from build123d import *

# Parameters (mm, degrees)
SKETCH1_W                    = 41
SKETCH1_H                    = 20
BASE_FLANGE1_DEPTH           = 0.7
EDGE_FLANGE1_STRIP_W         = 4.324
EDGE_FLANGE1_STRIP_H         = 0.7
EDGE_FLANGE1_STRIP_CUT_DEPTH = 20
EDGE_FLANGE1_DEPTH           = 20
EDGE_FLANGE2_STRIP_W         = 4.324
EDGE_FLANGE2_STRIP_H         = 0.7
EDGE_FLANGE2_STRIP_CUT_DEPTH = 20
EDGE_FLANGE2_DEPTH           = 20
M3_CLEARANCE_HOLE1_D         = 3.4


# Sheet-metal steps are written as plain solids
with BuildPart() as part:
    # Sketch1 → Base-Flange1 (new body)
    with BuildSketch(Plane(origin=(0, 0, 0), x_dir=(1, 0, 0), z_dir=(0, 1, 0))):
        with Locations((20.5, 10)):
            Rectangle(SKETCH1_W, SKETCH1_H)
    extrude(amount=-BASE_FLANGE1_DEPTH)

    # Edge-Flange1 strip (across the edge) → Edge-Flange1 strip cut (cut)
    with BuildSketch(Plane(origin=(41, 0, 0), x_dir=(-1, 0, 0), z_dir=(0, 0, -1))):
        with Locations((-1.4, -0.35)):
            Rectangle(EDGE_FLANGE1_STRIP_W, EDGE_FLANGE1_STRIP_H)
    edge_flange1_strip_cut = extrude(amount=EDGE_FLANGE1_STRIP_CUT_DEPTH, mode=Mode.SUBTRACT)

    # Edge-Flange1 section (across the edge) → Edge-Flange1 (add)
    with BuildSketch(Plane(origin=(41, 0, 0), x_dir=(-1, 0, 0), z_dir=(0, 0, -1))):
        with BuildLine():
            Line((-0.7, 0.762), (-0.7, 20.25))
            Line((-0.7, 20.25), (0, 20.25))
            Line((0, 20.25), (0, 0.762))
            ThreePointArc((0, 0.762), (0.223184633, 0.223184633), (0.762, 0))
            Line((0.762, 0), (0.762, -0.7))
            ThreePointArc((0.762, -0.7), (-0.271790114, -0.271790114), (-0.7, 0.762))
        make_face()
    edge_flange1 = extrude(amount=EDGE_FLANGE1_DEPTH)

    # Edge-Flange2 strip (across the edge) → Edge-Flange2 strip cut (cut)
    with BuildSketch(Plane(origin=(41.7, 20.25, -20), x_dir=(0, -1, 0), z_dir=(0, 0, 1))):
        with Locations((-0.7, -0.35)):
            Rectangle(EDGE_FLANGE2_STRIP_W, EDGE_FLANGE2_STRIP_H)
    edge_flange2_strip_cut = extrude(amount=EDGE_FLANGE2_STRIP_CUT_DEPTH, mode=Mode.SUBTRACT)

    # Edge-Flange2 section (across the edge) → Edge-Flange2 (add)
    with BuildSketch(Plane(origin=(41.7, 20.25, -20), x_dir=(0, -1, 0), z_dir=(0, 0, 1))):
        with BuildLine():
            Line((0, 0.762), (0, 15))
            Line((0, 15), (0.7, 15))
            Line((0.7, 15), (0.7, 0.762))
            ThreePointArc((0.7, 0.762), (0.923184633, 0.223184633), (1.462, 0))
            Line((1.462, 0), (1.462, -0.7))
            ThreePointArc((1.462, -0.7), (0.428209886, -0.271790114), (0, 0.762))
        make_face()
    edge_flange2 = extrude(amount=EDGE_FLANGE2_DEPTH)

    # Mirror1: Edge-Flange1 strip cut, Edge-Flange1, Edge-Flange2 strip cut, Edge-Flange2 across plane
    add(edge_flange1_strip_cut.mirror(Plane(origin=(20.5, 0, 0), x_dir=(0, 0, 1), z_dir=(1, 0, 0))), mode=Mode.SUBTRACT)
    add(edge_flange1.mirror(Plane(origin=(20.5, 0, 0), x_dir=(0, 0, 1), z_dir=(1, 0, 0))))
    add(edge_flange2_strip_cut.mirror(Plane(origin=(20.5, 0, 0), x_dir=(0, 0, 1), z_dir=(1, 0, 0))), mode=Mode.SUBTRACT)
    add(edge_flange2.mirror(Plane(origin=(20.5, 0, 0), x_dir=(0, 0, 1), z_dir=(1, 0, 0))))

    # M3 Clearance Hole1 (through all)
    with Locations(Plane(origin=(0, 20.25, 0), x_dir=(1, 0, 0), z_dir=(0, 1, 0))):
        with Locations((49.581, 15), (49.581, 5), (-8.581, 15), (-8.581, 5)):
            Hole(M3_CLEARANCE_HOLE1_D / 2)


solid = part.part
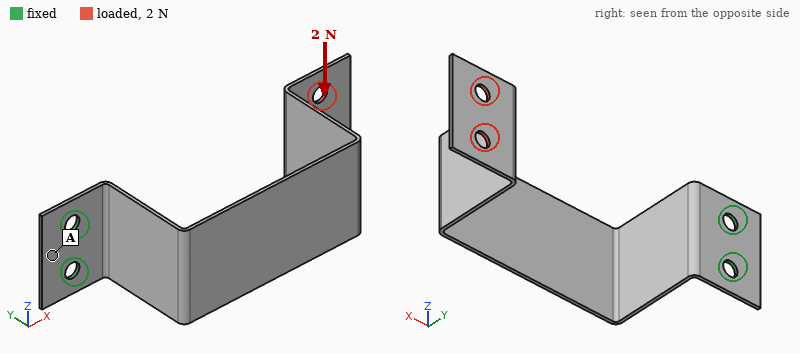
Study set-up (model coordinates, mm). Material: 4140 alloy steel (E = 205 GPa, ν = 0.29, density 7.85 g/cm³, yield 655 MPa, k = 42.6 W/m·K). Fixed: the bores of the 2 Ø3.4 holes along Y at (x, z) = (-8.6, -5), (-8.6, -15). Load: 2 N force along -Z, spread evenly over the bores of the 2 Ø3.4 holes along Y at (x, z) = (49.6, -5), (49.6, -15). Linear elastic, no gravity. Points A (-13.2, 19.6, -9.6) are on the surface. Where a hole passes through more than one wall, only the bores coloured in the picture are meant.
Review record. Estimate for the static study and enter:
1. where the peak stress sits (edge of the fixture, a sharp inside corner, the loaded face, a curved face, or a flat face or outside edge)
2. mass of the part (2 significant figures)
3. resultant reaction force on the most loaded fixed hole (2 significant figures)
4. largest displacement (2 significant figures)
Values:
a curved face
12 g
9.5 N
0.75 mm
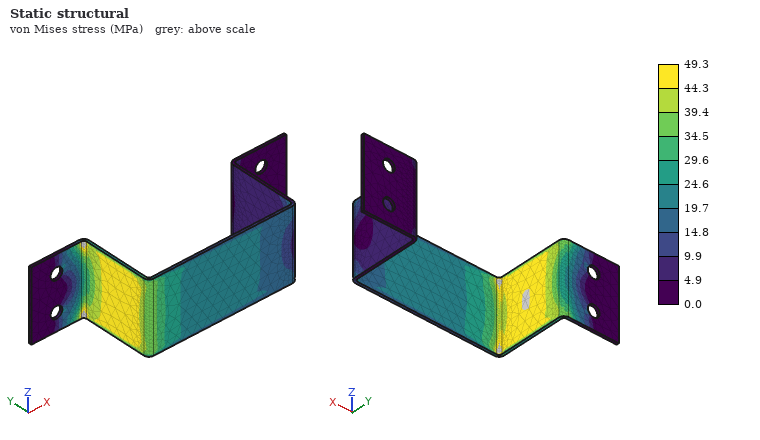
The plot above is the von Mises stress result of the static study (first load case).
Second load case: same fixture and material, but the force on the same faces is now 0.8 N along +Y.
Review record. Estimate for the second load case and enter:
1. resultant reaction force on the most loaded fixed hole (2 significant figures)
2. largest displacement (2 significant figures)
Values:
0.66 N
0.88 mm
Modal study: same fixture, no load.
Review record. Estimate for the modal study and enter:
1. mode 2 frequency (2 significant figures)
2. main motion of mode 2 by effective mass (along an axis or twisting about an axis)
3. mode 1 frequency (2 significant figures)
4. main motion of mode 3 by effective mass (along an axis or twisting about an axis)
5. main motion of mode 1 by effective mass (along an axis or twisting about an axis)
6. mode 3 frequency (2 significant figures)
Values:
150 Hz
along Z
82 Hz
along X
along Y
270 Hz
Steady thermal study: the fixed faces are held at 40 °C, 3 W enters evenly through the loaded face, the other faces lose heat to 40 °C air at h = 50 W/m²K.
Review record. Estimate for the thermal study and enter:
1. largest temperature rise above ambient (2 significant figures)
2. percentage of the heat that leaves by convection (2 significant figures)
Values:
66 K
99 %
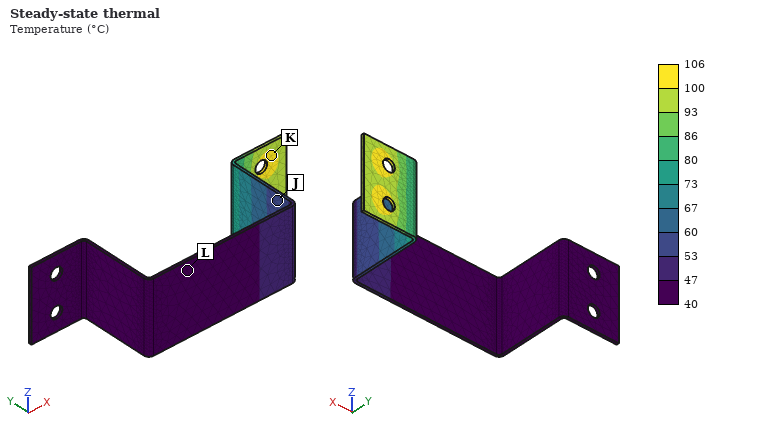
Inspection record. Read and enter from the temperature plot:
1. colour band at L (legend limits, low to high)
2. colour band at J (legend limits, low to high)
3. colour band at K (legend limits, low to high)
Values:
40 to 47 °C
53 to 60 °C
100 to 106 °C
